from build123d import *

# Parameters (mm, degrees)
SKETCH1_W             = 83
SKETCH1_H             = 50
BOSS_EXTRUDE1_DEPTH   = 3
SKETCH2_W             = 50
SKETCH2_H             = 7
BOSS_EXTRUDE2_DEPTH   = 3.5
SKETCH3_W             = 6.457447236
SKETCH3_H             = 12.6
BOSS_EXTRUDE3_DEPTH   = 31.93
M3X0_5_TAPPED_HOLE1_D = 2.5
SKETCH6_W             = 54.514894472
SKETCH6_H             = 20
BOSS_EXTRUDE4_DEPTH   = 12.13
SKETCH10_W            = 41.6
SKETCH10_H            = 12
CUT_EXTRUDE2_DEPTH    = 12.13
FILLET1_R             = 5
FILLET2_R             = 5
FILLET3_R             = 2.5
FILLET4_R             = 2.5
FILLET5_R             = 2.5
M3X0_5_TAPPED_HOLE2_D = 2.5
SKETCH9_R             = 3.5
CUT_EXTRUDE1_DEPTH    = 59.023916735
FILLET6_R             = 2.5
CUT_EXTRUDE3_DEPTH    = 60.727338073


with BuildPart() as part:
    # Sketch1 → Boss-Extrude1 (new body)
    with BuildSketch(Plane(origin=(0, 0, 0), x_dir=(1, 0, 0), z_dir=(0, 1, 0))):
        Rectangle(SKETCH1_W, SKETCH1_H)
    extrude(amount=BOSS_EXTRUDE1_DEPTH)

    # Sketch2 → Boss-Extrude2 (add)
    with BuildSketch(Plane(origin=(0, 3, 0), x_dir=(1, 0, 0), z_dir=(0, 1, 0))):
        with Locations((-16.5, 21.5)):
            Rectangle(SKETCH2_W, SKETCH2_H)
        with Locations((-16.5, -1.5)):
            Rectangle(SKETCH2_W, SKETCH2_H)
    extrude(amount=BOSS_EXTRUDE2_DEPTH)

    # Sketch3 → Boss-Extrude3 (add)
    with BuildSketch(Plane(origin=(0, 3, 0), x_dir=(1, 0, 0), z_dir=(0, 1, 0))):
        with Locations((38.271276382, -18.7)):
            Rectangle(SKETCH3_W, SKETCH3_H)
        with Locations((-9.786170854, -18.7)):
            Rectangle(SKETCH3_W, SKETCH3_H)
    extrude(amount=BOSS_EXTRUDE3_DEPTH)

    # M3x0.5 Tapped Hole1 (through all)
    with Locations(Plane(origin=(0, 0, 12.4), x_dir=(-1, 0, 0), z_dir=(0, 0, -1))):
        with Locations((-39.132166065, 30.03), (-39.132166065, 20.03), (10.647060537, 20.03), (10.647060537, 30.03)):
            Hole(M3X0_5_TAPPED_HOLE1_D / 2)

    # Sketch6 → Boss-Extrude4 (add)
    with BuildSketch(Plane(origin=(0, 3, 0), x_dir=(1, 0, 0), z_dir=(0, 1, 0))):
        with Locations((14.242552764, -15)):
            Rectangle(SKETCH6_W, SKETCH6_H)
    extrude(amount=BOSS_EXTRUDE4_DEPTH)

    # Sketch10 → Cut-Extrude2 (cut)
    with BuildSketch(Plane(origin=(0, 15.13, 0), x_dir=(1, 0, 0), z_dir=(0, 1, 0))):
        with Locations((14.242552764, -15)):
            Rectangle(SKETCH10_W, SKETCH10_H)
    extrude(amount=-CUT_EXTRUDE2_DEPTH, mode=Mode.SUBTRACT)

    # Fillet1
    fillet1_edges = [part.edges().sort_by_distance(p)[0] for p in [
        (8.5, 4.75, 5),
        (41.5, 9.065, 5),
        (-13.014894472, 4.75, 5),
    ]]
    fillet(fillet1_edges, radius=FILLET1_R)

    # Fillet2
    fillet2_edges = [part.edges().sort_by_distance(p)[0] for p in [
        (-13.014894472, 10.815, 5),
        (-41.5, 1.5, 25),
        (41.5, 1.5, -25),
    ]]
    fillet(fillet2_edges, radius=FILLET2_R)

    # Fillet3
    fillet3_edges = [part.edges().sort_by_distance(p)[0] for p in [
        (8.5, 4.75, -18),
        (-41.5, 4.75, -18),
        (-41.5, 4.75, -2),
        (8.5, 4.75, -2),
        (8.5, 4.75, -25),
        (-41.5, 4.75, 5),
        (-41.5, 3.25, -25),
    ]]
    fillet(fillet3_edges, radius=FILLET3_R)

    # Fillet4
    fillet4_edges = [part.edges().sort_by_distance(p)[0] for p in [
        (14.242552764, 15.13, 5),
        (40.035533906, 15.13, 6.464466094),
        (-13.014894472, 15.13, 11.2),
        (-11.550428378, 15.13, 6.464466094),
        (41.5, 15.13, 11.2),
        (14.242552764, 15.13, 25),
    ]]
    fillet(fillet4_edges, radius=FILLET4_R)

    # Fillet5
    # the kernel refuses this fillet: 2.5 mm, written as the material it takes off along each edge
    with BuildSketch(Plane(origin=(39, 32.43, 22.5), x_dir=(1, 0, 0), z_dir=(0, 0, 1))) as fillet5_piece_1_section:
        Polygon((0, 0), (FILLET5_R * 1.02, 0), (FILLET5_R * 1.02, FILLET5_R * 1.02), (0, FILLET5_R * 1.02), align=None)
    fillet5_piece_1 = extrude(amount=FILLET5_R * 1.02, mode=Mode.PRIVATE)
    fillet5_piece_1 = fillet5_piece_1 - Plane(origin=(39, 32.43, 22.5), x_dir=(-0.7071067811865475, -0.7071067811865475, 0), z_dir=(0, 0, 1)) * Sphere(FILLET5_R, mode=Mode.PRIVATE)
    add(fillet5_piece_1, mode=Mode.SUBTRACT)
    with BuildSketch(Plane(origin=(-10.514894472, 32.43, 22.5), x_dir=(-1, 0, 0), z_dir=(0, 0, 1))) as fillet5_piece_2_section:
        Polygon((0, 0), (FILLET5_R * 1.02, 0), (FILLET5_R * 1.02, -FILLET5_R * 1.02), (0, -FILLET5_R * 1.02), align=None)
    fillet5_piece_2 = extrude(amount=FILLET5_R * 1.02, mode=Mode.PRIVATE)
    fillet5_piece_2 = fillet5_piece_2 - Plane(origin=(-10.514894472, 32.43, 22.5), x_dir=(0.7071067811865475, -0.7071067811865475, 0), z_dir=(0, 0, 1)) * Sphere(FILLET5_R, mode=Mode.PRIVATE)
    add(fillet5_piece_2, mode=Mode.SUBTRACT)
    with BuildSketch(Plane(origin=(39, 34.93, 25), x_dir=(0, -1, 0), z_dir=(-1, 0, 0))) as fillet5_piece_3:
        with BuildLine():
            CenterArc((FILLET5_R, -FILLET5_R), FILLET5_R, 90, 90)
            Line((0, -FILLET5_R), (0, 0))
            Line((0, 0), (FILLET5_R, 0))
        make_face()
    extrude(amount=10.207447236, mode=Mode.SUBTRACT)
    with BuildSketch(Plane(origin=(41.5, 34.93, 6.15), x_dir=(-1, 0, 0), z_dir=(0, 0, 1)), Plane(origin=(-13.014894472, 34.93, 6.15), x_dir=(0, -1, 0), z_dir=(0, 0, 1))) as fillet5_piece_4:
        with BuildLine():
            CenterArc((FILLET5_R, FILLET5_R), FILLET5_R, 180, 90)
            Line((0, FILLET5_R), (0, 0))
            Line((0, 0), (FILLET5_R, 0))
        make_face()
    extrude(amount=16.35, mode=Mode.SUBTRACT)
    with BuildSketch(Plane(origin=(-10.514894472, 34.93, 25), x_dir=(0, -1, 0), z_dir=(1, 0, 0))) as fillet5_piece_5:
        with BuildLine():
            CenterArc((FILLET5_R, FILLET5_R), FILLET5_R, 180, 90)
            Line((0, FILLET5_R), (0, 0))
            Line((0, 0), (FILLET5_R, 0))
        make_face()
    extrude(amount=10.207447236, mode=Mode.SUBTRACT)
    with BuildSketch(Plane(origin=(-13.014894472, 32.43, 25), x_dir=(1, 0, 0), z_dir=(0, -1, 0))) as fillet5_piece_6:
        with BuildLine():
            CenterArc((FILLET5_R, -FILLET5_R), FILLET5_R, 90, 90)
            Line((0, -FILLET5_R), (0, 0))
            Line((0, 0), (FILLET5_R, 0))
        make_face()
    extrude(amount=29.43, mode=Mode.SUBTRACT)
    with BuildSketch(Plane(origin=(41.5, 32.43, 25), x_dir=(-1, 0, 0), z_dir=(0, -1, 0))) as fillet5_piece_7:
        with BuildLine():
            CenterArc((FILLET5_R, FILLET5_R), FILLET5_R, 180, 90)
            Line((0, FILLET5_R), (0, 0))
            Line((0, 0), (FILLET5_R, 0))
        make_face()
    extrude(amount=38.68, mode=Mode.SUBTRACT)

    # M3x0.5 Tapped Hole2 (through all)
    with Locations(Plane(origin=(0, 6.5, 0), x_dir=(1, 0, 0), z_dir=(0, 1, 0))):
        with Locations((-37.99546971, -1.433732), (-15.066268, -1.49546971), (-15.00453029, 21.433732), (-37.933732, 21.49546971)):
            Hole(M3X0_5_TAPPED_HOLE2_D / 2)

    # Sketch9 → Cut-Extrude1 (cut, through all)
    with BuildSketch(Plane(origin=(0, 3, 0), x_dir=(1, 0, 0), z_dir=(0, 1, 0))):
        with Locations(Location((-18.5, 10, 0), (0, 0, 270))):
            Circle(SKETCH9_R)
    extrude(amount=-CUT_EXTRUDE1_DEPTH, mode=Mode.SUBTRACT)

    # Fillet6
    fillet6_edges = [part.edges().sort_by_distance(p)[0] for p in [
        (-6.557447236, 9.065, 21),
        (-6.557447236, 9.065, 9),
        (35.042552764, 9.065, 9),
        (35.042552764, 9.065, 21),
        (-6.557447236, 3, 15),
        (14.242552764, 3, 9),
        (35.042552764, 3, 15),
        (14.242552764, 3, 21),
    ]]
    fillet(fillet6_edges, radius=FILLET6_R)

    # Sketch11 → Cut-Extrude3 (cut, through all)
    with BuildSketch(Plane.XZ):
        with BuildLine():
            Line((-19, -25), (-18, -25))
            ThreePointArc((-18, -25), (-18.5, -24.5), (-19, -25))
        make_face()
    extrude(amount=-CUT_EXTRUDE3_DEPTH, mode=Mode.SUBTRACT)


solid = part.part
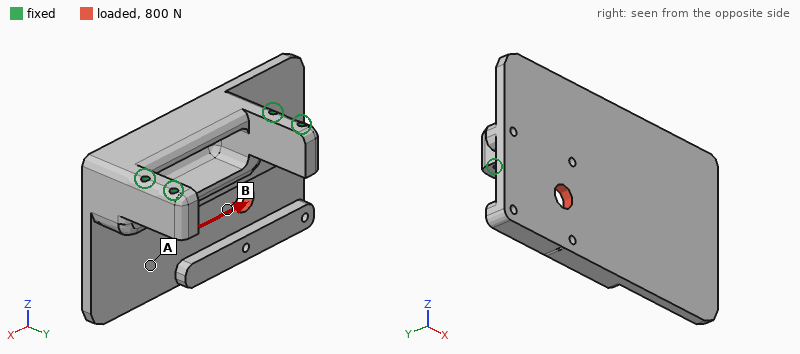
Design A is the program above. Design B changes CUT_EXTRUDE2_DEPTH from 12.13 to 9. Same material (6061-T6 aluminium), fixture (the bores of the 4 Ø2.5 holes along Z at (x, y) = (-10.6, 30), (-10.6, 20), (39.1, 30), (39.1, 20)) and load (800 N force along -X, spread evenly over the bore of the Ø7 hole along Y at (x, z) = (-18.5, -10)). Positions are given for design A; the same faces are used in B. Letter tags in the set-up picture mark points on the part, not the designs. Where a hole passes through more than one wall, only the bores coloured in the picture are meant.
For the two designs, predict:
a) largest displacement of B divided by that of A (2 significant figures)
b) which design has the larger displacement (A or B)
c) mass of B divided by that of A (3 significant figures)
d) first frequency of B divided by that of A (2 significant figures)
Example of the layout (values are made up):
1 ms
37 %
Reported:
0.88
A
1.06
1.0
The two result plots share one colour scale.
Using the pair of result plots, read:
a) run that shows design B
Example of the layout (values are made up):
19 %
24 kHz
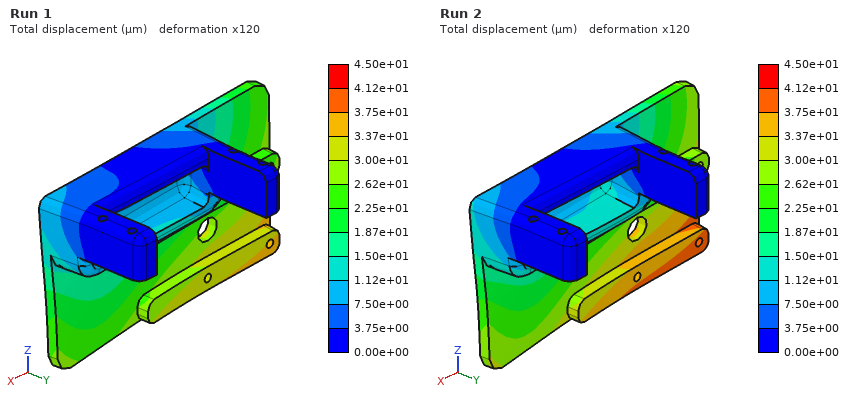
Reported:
Run 1
